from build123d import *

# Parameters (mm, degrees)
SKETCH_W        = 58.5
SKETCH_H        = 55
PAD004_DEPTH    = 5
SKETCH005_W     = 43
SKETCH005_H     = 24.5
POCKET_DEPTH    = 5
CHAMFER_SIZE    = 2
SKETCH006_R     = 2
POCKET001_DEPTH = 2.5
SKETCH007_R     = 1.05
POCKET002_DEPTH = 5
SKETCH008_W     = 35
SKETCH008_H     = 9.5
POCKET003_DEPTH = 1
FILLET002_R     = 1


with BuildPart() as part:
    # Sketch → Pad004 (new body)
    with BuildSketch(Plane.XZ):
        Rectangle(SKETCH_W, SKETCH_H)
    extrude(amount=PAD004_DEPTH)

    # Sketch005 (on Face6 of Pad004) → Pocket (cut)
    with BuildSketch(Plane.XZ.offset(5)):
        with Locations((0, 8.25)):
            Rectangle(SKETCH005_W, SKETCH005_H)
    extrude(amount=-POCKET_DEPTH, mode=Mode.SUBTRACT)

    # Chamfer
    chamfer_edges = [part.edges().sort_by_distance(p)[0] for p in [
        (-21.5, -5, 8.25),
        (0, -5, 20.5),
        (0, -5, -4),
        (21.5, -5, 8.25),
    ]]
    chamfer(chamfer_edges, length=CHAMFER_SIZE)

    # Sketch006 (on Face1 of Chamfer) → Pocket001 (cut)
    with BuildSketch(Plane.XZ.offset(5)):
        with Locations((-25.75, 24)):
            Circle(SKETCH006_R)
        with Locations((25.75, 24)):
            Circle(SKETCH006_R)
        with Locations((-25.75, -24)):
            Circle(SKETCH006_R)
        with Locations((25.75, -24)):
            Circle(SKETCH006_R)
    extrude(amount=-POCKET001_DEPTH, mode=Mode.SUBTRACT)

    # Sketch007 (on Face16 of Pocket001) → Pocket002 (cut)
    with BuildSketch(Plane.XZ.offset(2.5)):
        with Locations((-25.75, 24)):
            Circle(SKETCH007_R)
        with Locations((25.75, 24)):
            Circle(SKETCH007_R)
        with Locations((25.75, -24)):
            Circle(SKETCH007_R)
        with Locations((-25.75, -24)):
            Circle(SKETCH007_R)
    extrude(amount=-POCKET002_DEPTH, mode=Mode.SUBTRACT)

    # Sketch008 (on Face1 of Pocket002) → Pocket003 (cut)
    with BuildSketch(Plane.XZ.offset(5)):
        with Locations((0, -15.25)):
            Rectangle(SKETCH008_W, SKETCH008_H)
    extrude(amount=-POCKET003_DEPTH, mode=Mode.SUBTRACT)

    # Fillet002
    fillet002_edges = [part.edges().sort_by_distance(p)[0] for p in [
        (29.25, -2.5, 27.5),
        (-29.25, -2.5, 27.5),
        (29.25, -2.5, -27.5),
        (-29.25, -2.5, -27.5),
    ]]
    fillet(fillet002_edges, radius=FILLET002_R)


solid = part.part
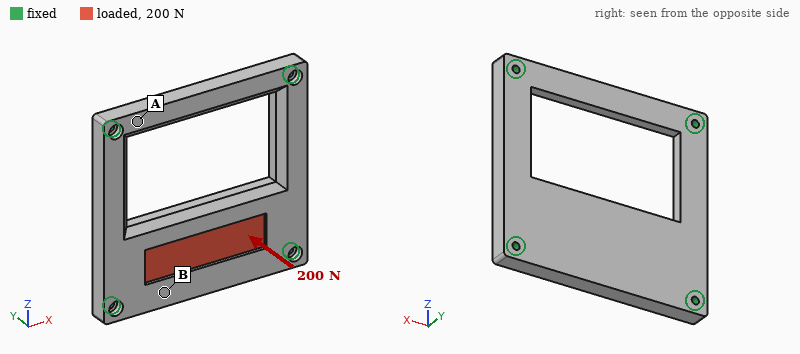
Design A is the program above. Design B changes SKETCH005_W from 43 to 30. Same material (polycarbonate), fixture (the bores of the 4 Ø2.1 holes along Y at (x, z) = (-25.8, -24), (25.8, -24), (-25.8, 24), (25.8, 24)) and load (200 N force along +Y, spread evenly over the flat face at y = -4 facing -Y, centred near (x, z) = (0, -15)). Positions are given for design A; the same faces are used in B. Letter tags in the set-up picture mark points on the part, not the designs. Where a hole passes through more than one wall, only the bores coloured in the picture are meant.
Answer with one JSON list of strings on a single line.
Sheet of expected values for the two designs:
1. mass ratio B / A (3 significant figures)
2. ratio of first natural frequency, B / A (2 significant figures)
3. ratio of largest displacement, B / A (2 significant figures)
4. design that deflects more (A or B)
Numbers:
["1.16", "1.0", "0.76", "A"]
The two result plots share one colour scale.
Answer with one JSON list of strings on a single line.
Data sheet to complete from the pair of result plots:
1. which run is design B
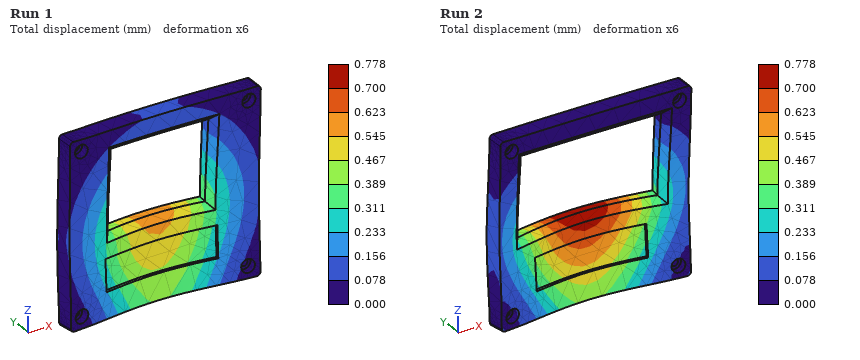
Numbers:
["Run 1"]
